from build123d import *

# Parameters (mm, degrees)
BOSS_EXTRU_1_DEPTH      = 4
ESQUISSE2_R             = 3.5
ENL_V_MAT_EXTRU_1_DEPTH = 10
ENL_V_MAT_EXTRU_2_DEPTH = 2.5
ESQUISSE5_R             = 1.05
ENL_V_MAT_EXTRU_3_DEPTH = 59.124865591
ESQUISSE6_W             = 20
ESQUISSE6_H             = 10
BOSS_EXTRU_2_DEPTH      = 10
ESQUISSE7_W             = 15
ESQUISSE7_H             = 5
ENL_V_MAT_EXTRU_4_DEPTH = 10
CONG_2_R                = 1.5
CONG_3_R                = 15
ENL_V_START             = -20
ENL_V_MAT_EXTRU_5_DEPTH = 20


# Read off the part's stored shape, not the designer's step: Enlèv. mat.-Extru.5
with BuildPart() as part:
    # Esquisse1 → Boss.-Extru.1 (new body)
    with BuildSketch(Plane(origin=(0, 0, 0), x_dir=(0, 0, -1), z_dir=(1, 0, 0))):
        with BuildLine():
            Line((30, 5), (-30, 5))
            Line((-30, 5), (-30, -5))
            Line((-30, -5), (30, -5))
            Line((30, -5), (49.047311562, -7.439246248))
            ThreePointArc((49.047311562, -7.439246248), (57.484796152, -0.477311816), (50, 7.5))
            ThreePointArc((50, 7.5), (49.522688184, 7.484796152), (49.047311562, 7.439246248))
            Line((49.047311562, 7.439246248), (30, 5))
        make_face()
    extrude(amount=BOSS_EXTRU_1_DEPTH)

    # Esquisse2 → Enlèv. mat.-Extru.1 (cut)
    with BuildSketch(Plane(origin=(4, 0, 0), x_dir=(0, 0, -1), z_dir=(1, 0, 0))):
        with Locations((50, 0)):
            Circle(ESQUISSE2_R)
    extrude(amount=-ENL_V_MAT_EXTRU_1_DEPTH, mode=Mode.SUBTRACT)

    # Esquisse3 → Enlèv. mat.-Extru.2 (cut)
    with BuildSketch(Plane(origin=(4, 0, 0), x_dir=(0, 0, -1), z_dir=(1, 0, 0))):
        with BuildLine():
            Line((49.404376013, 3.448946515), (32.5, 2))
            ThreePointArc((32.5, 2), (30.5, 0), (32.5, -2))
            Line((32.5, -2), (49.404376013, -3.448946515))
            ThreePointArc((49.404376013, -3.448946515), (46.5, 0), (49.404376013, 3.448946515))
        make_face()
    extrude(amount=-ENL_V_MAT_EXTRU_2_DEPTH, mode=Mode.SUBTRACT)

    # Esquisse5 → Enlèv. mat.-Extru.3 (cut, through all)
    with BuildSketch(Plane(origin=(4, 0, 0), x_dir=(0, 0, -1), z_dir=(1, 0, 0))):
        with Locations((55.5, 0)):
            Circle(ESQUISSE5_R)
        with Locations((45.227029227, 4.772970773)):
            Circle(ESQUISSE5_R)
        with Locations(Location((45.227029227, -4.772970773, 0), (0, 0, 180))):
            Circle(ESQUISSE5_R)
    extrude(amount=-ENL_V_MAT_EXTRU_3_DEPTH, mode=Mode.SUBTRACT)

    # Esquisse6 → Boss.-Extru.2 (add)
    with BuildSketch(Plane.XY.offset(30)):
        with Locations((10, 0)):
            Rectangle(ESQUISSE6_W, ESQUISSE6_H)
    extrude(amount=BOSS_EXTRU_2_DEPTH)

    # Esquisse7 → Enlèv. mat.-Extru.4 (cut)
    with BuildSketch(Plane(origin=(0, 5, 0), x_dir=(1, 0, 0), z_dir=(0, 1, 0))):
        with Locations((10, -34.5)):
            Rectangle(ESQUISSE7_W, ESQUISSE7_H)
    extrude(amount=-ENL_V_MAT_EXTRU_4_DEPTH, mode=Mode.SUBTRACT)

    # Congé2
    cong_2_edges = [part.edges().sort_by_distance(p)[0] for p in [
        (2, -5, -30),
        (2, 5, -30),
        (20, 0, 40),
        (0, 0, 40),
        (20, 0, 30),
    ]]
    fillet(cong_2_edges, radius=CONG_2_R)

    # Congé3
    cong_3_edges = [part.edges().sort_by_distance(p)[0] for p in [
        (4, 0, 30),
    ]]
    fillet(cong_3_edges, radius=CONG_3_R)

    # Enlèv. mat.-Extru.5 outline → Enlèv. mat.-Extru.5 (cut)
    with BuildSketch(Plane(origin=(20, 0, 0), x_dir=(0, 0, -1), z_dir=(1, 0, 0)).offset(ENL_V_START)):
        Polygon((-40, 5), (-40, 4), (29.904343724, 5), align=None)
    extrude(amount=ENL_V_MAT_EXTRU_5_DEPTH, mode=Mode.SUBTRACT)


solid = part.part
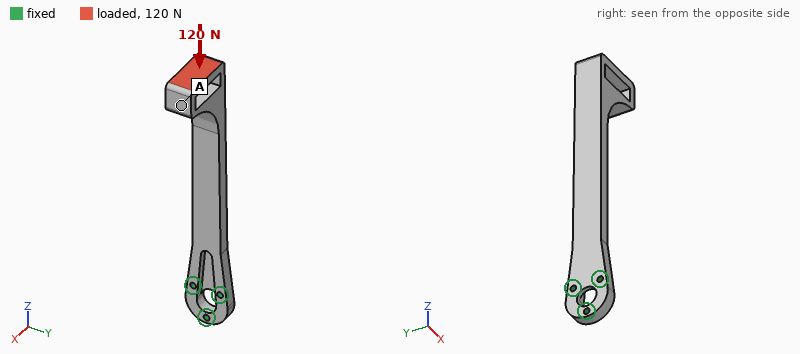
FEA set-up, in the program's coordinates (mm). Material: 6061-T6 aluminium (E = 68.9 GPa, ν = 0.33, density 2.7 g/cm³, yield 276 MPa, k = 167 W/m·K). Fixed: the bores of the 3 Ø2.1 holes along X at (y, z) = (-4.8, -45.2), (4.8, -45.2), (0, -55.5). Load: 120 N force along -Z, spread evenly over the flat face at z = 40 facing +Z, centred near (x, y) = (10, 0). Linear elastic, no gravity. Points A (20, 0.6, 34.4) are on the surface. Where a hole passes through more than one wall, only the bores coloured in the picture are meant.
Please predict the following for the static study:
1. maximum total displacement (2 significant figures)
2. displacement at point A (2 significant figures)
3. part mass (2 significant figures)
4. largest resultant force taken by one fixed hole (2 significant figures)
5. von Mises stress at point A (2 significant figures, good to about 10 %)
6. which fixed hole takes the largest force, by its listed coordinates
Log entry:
1.0 mm
0.93 mm
13 g
66 N
9.0 MPa
(-4.8, -45.2)
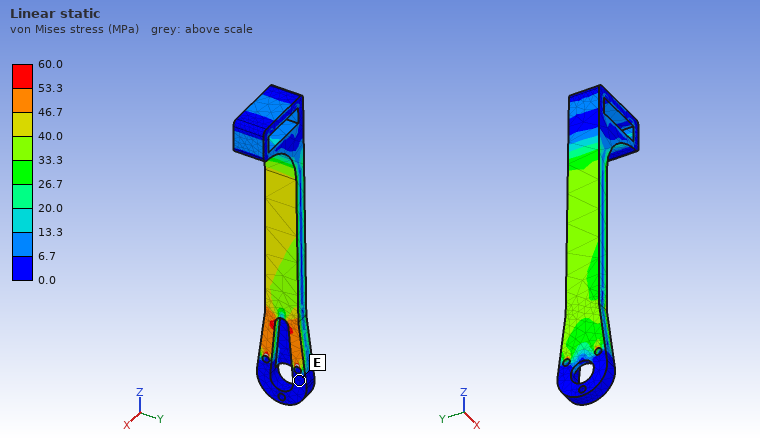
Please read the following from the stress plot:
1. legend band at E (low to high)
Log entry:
0.0 to 6.7 MPa
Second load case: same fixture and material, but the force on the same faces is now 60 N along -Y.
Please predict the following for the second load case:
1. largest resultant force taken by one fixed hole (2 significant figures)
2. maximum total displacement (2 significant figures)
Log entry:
490 N
0.61 mm
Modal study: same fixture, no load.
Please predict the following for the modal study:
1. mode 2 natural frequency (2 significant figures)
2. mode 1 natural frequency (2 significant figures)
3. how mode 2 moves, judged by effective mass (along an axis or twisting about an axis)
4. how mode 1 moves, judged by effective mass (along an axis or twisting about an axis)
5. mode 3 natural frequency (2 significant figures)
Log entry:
830 Hz
300 Hz
along Y
along X
2200 Hz
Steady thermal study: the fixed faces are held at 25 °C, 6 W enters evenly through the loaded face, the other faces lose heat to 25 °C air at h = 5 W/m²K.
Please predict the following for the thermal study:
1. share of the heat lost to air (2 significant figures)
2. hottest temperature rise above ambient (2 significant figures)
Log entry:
11 %
72 K
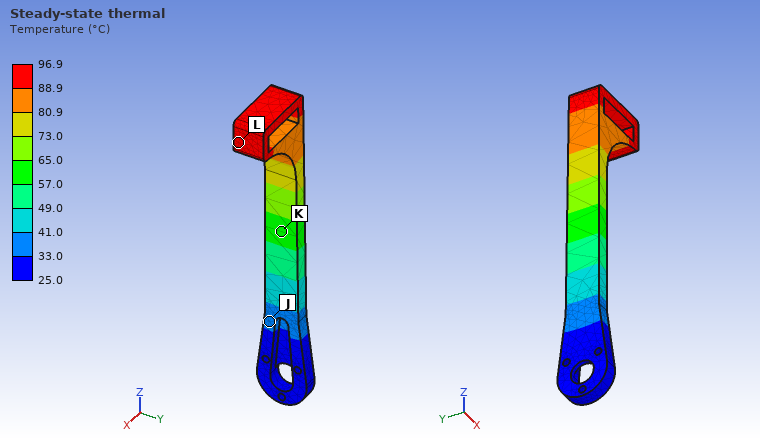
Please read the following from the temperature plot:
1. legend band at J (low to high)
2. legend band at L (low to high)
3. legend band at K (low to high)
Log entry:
33.0 to 41.0 °C
88.9 to 96.9 °C
57.0 to 65.0 °C
